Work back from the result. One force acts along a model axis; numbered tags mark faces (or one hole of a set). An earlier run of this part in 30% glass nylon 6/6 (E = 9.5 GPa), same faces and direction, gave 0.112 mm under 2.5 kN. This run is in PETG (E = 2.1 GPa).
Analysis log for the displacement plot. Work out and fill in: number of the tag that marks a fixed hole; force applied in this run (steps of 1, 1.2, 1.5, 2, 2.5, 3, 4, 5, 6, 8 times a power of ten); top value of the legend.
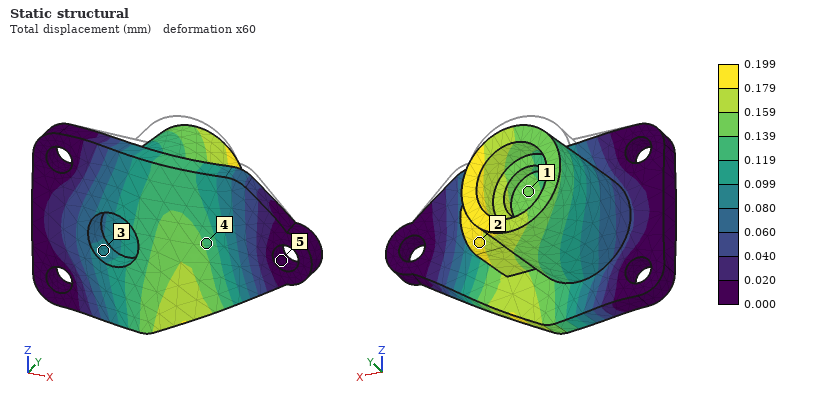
5
1 kN
0.199 mm
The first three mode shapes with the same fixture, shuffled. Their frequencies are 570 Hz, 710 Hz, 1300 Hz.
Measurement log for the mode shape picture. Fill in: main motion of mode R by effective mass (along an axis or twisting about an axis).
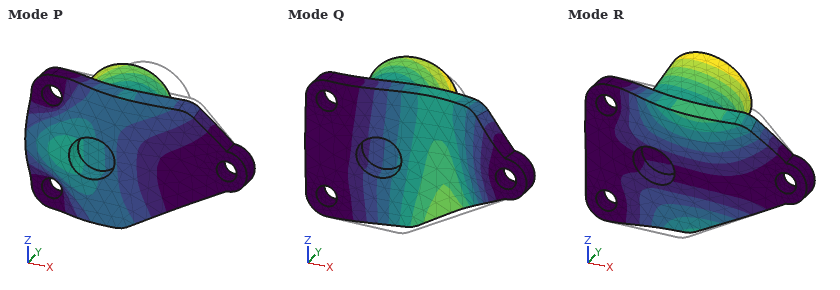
along Z
